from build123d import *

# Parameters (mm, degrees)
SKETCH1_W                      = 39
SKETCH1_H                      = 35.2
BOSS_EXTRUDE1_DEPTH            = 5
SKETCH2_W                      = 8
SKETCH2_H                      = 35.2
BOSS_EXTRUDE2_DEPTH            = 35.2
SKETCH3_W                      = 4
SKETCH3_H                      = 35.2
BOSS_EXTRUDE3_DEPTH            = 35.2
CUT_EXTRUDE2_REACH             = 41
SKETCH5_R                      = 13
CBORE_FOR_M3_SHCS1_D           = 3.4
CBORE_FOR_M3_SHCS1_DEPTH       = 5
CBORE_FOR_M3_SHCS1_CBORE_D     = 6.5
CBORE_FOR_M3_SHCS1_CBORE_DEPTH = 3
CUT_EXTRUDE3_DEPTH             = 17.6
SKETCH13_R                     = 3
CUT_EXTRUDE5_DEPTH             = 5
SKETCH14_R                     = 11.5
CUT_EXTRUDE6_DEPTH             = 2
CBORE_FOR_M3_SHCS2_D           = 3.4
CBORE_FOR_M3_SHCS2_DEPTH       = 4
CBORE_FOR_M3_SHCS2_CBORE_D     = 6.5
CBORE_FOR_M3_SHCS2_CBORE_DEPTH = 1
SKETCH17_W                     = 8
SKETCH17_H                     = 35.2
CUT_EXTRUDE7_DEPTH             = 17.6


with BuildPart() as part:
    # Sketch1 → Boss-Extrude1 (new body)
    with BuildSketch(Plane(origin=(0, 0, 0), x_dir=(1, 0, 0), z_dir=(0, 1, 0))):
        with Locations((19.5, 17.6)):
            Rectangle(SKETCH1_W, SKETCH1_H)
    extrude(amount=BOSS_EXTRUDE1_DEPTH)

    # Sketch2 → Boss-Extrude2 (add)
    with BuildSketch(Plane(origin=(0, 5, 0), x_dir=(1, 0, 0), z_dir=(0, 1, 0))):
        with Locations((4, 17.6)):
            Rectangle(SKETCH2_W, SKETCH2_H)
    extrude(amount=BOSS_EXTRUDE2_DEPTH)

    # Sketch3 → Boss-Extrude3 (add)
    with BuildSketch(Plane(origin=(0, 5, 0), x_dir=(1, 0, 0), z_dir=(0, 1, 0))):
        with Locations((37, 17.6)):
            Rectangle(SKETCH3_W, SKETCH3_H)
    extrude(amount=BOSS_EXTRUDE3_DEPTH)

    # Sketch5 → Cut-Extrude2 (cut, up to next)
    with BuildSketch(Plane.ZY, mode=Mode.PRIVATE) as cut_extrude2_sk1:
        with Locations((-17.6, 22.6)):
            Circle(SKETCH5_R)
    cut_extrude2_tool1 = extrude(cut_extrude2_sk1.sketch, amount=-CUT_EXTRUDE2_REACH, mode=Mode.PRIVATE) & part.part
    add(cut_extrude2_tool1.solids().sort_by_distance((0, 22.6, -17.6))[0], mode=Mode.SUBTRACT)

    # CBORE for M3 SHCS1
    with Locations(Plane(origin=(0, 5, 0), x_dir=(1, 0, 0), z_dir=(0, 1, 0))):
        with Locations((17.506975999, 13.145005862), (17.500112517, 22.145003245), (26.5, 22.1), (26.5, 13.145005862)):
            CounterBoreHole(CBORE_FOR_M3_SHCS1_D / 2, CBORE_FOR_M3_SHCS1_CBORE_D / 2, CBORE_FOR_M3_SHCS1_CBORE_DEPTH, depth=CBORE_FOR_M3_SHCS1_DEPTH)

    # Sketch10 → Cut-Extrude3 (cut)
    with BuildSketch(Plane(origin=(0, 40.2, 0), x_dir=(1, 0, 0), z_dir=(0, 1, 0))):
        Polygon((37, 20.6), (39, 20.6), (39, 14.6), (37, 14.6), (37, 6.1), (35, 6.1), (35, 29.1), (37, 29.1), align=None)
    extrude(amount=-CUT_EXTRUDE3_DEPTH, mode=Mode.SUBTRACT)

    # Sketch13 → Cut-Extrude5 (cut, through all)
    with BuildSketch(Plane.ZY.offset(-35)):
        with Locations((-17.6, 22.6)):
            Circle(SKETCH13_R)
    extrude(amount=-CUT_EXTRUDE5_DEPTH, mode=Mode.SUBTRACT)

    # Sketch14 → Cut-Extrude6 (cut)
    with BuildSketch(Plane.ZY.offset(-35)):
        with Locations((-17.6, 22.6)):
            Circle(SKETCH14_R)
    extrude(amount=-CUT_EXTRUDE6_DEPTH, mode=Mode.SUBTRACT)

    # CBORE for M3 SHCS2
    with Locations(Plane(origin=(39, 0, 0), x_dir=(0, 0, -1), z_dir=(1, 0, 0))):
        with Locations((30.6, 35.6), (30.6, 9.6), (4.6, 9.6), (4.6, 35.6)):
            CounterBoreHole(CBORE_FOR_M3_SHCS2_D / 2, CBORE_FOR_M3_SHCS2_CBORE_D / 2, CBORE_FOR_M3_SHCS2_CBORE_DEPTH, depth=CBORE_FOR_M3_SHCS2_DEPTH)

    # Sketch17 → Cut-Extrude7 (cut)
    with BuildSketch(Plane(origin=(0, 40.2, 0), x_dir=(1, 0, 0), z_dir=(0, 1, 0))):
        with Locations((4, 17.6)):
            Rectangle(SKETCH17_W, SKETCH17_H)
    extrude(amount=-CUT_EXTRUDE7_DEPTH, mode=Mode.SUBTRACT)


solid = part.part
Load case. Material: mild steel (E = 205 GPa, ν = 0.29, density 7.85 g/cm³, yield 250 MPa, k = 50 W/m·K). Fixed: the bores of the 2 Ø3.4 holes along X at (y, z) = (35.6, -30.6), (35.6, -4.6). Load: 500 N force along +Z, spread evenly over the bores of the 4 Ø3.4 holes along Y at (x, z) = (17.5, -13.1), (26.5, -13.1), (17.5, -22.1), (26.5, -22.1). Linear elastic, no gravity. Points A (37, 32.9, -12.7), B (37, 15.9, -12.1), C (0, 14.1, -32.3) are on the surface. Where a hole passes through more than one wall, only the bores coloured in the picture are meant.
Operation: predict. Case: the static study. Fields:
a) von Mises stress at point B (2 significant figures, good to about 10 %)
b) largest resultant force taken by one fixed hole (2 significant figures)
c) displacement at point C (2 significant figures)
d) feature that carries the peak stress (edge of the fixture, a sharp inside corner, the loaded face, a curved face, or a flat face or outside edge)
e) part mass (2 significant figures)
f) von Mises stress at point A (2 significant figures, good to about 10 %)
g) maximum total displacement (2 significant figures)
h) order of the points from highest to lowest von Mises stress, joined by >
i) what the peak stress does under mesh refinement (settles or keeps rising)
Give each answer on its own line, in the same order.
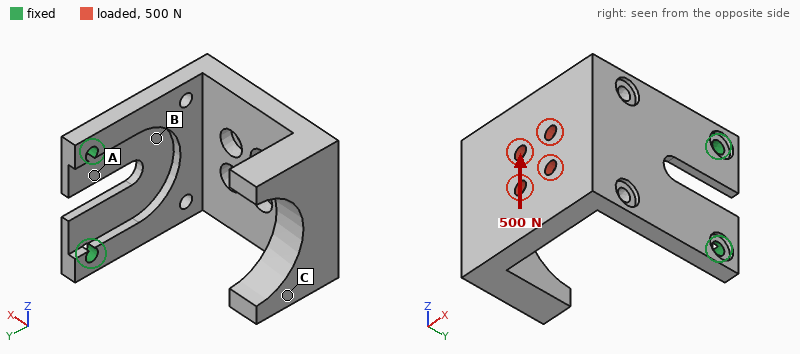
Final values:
65 MPa
620 N
0.22 mm
edge of the fixture
98 g
33 MPa
0.23 mm
B > A > C
keeps rising
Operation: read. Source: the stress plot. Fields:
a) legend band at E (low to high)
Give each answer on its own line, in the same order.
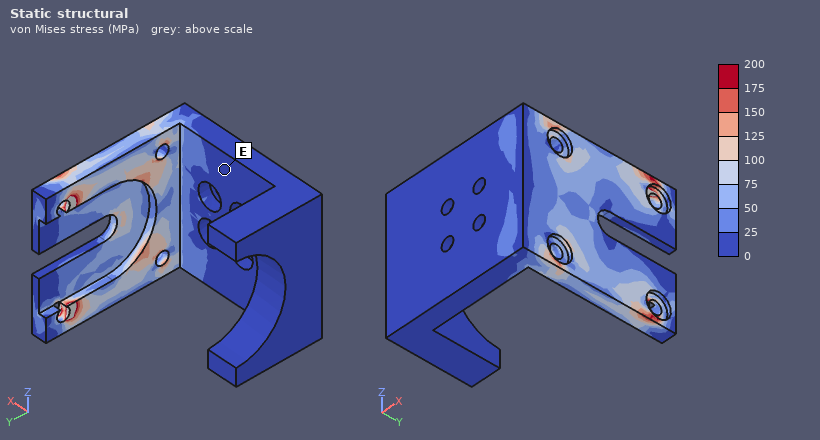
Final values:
0 to 25 MPa
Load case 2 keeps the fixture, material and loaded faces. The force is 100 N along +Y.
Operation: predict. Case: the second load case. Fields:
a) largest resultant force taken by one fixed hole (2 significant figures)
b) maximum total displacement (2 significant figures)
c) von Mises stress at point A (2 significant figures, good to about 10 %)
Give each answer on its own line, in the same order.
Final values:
56 N
0.11 mm
11 MPa
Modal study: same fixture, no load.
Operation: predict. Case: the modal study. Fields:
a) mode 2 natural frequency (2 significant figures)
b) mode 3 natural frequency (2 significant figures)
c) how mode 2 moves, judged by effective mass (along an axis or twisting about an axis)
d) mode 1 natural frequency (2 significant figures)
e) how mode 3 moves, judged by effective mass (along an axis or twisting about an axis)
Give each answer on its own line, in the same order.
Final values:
780 Hz
1500 Hz
along Z
460 Hz
along X
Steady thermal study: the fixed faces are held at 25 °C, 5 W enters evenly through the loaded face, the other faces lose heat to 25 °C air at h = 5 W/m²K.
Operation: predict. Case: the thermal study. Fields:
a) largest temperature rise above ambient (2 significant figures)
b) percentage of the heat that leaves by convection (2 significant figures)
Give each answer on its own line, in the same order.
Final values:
40 K
21 %
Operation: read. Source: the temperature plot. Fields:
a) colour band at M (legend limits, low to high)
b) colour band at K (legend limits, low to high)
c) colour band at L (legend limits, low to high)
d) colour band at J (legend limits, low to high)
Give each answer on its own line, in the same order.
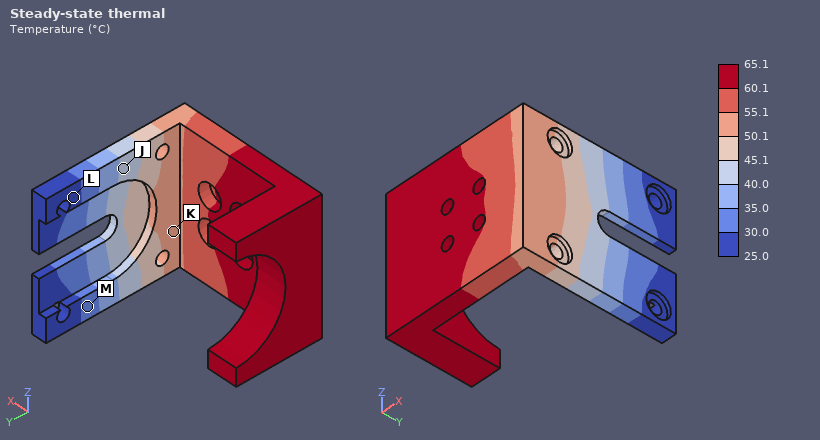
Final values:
30.0 to 35.0 °C
50.1 to 55.1 °C
25.0 to 30.0 °C
40.0 to 45.1 °C
